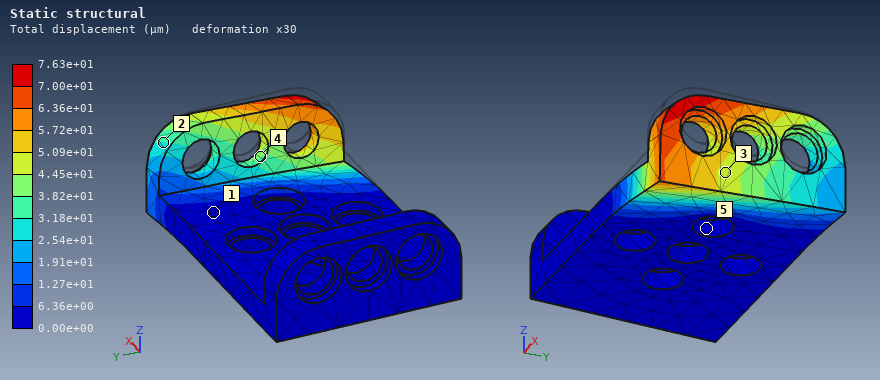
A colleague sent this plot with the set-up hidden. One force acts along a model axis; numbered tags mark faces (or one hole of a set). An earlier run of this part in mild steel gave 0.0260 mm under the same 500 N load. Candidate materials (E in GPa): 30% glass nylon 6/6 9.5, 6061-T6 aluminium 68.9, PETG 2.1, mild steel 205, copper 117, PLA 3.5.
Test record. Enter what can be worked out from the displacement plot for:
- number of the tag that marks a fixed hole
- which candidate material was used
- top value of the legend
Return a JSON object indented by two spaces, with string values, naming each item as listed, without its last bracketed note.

{
  "number of the tag that marks a fixed hole": "5",
  "which candidate material was used": "6061-T6 aluminium",
  "top value of the legend": "7.63e+01 µm"
}
